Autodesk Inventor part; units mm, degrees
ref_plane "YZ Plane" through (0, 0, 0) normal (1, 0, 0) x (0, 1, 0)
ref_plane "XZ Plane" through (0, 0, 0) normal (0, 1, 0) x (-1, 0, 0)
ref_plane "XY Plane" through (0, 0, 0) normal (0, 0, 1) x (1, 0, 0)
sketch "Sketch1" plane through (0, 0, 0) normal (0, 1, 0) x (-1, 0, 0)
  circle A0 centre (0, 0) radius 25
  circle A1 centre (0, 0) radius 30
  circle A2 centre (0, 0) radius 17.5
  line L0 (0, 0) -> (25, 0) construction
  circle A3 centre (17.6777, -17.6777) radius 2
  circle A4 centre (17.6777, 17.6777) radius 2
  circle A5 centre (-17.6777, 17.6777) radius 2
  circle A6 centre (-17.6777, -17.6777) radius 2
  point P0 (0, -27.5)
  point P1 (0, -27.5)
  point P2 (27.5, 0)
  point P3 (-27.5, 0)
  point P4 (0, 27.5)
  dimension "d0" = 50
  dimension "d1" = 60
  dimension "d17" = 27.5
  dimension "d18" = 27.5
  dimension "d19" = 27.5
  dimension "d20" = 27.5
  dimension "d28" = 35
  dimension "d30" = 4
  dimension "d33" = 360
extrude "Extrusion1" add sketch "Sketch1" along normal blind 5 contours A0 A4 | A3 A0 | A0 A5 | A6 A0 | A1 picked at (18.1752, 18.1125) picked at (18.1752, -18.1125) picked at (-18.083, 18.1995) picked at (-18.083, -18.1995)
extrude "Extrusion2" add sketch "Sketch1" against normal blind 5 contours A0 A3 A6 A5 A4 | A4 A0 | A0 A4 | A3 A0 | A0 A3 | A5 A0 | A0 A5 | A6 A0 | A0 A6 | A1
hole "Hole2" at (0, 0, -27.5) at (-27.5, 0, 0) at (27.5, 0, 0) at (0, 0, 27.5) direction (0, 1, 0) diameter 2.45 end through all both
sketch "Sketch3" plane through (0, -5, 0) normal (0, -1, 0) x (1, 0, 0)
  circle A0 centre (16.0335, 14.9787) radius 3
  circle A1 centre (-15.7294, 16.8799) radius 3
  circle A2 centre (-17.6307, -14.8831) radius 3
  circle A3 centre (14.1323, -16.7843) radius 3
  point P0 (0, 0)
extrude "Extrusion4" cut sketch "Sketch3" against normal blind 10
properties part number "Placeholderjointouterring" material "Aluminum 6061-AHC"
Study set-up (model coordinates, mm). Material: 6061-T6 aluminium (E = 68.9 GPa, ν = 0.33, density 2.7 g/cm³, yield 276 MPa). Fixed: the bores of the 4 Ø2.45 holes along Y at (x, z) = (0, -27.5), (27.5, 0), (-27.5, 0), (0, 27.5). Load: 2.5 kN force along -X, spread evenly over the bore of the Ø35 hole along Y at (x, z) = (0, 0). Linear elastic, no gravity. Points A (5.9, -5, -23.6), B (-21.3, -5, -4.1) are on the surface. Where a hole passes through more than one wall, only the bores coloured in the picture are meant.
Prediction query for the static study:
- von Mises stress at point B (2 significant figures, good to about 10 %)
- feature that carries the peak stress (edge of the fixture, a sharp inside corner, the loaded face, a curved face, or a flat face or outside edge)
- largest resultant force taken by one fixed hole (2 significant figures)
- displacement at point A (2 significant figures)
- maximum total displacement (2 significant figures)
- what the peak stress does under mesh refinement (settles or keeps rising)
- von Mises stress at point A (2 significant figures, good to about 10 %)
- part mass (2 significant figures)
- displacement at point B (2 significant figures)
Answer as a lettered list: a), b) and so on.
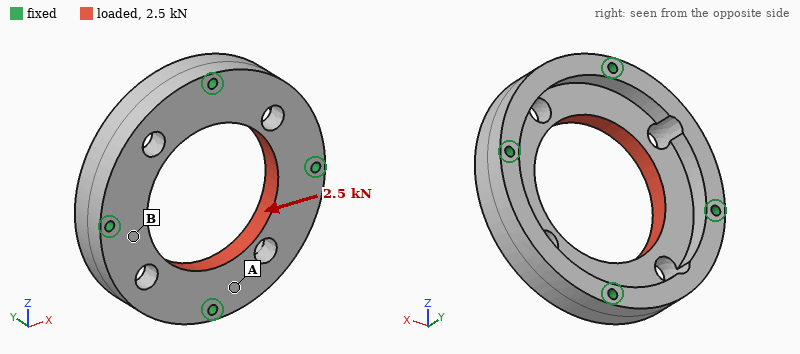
a) 10 MPa
b) edge of the fixture
c) 720 N
d) 2.0 µm
e) 5.0 µm
f) keeps rising
g) 4.1 MPa
h) 35 g
i) 1.7 µm
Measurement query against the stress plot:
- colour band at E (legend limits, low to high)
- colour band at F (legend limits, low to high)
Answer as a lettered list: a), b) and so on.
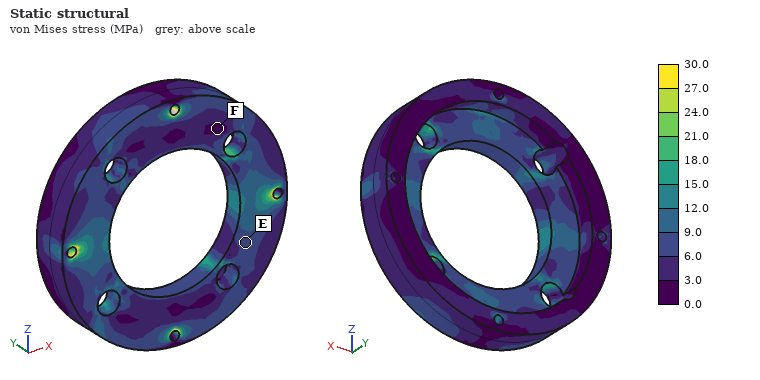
a) 6.0 to 9.0 MPa
b) 0.0 to 3.0 MPa
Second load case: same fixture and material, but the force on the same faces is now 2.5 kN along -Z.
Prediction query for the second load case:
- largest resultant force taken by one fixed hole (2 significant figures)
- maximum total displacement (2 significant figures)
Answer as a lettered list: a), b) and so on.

a) 730 N
b) 5.0 µm
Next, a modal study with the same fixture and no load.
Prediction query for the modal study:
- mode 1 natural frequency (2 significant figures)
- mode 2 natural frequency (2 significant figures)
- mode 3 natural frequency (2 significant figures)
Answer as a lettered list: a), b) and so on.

a) 19 kHz
b) 20 kHz
c) 20 kHz
